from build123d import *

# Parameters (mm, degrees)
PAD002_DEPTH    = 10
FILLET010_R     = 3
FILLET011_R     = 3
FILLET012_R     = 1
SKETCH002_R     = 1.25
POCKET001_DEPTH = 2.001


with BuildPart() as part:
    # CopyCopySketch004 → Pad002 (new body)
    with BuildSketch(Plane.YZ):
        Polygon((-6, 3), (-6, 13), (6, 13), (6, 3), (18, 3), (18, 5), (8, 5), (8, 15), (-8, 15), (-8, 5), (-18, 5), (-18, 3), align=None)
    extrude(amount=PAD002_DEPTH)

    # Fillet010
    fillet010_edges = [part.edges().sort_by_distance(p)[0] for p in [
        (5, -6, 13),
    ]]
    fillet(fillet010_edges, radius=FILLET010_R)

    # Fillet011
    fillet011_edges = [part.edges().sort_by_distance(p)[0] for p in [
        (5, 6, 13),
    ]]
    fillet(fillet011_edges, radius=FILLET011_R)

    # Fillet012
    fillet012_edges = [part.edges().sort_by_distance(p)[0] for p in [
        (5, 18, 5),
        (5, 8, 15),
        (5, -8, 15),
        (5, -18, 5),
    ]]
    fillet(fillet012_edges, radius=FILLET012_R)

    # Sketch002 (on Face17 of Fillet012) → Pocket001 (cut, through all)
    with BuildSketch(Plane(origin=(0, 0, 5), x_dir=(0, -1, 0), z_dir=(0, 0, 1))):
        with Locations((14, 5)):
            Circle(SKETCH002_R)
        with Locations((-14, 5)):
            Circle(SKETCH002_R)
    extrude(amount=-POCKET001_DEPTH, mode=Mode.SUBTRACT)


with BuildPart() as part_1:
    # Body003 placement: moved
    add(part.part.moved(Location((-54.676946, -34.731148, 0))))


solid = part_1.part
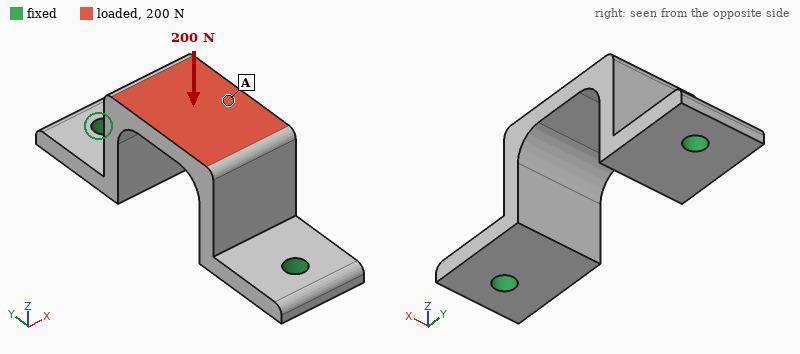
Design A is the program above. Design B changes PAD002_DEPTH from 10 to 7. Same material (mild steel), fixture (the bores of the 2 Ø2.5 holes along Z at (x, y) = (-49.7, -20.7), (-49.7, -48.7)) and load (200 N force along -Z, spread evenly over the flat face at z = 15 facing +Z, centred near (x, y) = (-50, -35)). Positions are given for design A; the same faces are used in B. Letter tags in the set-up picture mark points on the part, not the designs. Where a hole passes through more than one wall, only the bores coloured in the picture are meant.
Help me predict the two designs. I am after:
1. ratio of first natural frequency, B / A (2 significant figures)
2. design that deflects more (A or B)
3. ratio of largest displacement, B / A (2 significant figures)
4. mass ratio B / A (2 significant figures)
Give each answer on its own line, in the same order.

0.96
B
1.9
0.69
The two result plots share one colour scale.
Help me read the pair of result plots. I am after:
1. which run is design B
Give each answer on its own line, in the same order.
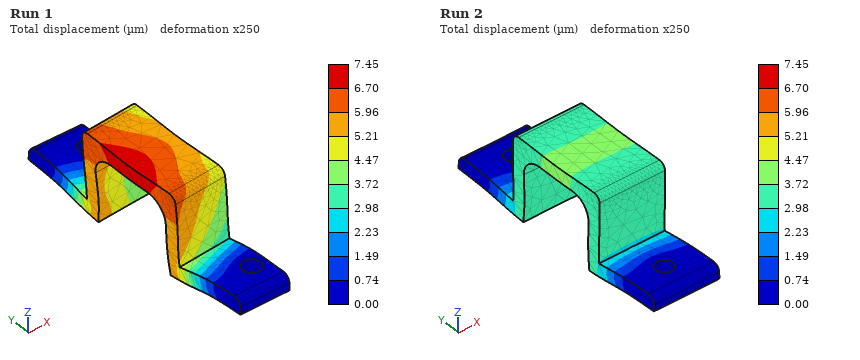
Run 1
